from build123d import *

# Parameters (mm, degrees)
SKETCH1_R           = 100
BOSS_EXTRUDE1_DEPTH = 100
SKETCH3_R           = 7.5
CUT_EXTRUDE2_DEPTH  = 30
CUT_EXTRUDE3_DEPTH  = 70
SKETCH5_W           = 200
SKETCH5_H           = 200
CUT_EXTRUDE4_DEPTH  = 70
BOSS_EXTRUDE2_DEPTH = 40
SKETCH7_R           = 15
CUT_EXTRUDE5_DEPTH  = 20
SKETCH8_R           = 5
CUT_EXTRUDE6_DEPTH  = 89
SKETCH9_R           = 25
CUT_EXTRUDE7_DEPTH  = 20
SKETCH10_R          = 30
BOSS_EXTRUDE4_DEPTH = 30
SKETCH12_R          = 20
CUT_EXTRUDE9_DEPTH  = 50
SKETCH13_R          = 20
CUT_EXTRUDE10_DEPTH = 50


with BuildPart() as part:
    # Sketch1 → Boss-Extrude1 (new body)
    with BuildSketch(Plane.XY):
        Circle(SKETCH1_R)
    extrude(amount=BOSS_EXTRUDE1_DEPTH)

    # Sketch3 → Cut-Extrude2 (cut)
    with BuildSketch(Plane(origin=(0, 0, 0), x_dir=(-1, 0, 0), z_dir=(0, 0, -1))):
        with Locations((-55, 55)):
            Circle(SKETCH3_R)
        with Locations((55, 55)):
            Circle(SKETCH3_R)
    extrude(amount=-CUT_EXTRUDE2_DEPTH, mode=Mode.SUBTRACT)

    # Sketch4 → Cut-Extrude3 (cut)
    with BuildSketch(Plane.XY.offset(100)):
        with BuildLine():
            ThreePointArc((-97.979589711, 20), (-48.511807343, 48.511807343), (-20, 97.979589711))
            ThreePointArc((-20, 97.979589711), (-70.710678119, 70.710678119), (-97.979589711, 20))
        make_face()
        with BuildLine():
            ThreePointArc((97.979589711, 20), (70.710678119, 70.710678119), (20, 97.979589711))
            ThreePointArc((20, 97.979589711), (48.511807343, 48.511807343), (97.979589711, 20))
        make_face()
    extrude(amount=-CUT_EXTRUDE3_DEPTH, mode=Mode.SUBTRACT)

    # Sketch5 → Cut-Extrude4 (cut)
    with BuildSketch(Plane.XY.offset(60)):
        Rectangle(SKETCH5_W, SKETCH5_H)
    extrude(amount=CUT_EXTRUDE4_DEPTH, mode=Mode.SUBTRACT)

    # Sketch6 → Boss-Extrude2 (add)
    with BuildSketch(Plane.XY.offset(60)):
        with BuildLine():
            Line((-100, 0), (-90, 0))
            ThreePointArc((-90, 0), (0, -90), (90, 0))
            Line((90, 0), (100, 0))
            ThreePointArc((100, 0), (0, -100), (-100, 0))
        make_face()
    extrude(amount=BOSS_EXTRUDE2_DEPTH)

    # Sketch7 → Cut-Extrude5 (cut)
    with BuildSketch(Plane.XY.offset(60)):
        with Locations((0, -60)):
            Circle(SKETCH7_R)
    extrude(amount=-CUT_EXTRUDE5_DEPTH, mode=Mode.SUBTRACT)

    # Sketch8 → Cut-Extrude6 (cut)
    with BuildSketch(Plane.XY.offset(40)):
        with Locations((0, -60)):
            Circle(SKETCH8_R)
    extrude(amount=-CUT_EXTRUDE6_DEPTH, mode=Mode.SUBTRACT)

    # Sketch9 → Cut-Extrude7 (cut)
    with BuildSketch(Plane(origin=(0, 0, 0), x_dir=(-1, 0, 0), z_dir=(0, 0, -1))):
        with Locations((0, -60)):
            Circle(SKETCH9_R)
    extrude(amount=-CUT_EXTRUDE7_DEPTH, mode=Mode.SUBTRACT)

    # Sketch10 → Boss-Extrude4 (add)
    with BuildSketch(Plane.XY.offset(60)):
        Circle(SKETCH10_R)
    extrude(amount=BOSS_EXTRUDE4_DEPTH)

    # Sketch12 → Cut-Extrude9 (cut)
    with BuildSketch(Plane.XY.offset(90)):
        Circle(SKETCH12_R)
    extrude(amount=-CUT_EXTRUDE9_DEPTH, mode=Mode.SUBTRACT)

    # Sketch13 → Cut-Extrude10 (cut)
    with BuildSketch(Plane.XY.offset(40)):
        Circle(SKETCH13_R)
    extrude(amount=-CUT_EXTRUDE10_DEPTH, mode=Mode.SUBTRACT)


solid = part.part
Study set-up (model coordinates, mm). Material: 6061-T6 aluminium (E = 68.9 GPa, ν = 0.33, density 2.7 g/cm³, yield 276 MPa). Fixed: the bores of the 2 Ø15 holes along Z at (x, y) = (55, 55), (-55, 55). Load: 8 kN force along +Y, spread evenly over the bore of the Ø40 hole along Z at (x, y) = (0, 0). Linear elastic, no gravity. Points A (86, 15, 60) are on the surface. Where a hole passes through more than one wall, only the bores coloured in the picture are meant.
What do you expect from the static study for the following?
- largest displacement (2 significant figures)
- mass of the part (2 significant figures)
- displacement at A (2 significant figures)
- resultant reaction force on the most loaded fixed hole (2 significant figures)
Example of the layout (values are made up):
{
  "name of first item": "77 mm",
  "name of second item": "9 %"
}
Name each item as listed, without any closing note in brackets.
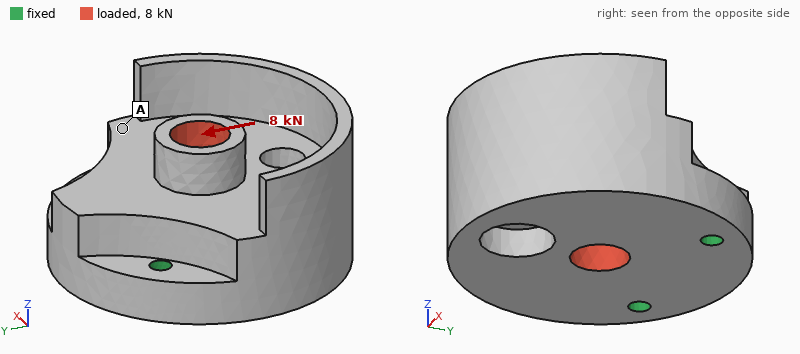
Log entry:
{
  "largest displacement": "43 µm",
  "mass of the part": "4.8 kg",
  "displacement at A": "13 µm",
  "resultant reaction force on the most loaded fixed hole": "4.0 kN"
}
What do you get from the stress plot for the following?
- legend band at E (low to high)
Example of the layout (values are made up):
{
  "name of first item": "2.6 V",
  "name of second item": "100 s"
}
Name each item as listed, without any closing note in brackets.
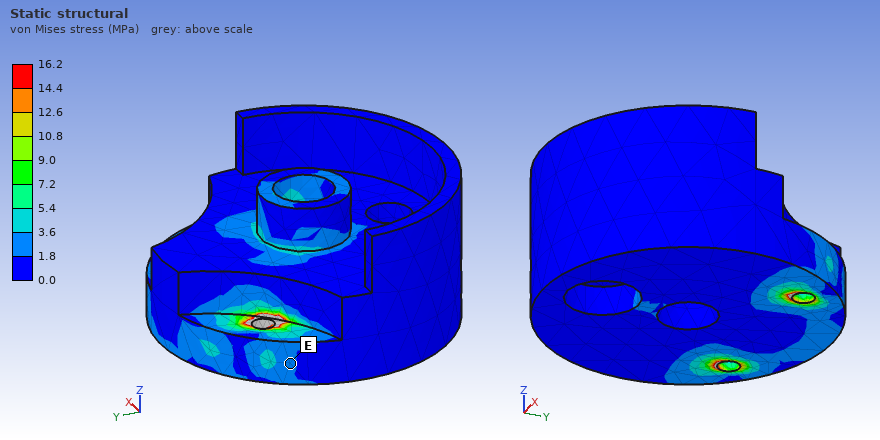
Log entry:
{
  "legend band at E": "1.8 to 3.6 MPa"
}
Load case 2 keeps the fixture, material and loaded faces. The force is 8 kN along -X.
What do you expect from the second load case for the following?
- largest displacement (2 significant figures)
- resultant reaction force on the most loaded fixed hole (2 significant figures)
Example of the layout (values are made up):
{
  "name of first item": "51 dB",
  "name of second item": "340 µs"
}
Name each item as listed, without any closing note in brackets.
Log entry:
{
  "largest displacement": "9.0 µm",
  "resultant reaction force on the most loaded fixed hole": "5.8 kN"
}
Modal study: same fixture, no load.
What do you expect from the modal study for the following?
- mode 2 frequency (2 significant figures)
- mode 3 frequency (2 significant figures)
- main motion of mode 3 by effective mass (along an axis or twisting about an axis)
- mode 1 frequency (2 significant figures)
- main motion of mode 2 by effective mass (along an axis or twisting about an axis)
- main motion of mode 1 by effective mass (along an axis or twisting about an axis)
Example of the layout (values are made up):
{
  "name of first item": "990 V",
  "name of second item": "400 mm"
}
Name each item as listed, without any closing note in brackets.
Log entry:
{
  "mode 2 frequency": "2400 Hz",
  "mode 3 frequency": "2600 Hz",
  "main motion of mode 3 by effective mass": "along X",
  "mode 1 frequency": "870 Hz",
  "main motion of mode 2 by effective mass": "along X",
  "main motion of mode 1 by effective mass": "along Z"
}
